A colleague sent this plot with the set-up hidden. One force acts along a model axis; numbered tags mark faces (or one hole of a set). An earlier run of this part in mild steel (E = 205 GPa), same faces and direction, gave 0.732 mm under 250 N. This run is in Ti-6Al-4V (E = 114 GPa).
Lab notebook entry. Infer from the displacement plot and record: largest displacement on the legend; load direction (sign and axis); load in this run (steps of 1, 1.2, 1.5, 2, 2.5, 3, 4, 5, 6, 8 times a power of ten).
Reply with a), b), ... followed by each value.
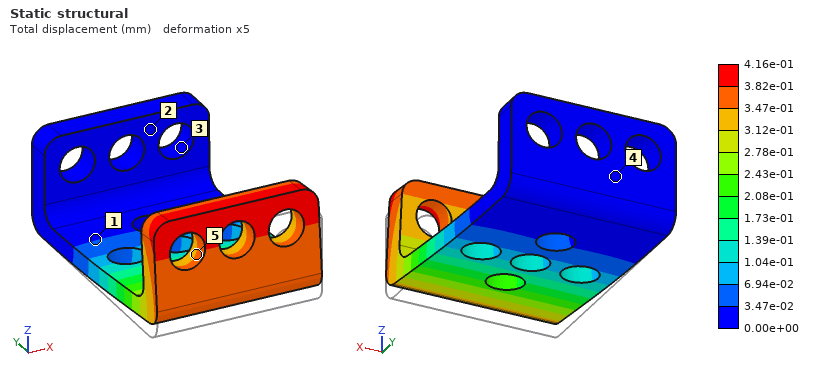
a) 4.16e-01 mm
b) +Z
c) 80 N
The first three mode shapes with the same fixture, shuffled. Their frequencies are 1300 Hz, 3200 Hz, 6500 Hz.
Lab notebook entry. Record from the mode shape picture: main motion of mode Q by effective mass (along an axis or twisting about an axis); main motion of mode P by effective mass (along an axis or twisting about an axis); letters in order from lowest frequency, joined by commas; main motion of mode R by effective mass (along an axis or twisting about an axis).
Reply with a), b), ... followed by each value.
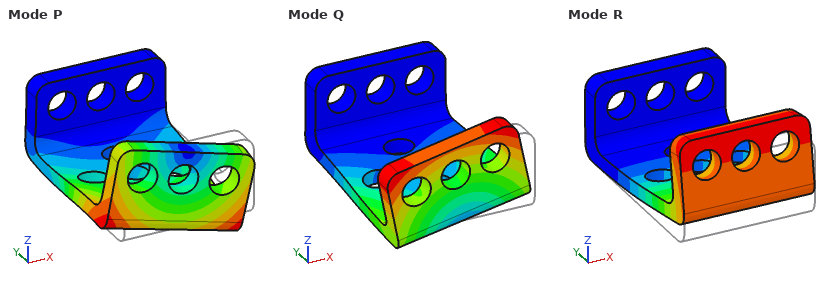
a) along X
b) along X
c) R, Q, P
d) along Z
